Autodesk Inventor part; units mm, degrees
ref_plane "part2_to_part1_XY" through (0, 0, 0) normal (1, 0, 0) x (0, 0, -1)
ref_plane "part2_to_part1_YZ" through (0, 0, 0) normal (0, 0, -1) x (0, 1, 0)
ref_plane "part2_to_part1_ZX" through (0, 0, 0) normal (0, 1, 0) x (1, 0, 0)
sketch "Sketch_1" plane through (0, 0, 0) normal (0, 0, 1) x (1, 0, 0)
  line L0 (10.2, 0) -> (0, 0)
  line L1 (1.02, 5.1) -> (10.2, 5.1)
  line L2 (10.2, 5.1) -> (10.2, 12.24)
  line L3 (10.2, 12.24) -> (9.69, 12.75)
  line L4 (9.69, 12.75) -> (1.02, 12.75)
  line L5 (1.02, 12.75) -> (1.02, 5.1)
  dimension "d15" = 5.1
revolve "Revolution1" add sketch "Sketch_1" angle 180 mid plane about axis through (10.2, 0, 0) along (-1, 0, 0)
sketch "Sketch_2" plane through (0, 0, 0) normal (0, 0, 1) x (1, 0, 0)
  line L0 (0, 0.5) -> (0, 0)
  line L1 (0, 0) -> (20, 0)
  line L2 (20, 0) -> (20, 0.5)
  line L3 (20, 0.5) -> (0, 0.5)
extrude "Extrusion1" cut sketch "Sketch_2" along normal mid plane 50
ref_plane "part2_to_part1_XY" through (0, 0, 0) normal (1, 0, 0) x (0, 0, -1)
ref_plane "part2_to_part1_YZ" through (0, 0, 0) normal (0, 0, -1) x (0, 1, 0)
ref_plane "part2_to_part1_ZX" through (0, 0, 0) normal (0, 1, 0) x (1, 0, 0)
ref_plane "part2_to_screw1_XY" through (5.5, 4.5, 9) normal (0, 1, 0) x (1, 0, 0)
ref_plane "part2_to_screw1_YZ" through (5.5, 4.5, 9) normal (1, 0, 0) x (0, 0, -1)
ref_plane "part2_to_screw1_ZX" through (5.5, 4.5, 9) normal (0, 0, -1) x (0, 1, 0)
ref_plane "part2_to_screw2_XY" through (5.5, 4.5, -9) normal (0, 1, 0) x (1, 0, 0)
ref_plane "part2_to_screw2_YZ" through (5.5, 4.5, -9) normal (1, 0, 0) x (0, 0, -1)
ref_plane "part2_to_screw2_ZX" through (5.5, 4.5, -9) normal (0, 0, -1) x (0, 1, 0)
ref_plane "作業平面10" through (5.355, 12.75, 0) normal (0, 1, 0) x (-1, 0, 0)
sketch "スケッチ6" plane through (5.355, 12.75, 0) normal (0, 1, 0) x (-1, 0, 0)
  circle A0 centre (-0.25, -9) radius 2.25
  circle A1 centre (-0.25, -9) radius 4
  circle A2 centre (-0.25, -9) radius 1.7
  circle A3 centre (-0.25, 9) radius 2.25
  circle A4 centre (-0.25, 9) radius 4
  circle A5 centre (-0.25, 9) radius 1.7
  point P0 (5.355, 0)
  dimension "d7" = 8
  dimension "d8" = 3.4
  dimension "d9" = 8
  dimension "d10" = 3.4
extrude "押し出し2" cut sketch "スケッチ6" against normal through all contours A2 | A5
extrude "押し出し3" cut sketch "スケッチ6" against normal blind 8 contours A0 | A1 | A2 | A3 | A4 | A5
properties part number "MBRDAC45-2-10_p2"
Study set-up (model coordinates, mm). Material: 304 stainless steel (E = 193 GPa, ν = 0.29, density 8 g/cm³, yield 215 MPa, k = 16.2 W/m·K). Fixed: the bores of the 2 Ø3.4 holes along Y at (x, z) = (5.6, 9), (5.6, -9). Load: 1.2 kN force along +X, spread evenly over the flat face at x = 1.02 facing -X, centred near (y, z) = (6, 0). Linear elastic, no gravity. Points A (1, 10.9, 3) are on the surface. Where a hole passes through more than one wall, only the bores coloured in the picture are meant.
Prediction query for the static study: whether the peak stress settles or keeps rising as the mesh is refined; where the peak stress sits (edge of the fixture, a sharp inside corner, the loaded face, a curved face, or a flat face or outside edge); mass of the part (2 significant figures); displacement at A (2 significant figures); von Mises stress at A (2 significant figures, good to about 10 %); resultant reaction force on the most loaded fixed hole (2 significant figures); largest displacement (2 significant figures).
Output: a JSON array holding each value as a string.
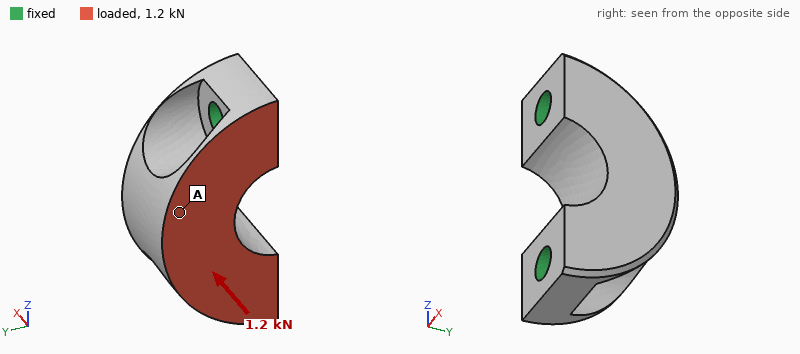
["keeps rising", "edge of the fixture", "11 g", "5.9 µm", "18 MPa", "600 N", "8.0 µm"]
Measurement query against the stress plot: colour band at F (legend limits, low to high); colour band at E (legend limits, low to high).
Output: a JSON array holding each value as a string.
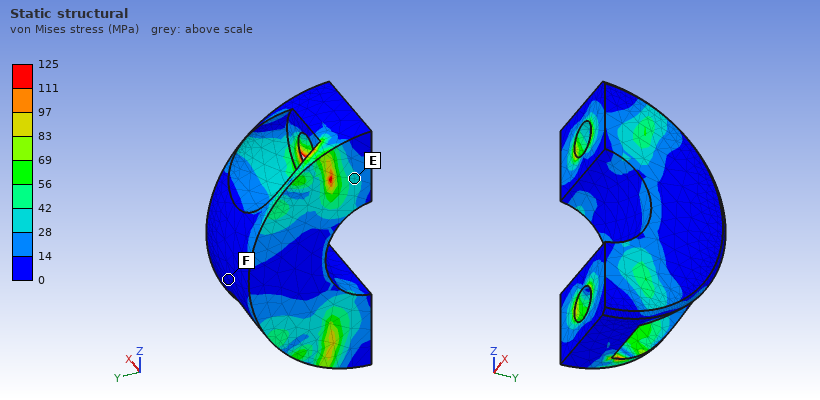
["0 to 14 MPa", "28 to 42 MPa"]
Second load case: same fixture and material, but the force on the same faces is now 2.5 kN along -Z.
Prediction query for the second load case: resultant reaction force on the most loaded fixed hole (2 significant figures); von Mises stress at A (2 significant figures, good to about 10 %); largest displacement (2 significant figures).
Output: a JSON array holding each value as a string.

["1.4 kN", "37 MPa", "7.4 µm"]
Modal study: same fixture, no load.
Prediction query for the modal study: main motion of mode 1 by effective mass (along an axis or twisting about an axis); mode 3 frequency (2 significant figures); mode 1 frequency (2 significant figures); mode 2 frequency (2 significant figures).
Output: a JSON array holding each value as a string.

["along X", "53 kHz", "23 kHz", "53 kHz"]
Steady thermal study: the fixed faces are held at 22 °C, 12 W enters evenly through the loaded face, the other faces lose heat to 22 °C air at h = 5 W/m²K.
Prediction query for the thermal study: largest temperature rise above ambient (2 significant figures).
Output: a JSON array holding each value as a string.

["66 K"]
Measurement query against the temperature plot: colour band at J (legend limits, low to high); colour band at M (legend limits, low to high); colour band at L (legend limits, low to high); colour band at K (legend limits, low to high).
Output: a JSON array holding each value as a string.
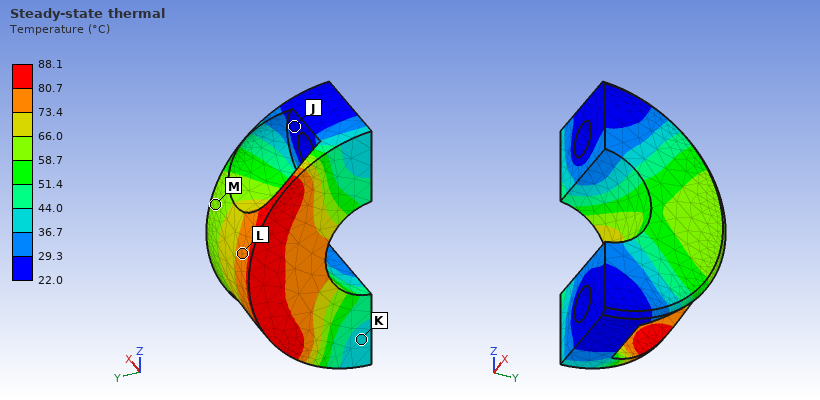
["22.0 to 29.3 °C", "58.7 to 66.0 °C", "73.4 to 80.7 °C", "36.7 to 44.0 °C"]
